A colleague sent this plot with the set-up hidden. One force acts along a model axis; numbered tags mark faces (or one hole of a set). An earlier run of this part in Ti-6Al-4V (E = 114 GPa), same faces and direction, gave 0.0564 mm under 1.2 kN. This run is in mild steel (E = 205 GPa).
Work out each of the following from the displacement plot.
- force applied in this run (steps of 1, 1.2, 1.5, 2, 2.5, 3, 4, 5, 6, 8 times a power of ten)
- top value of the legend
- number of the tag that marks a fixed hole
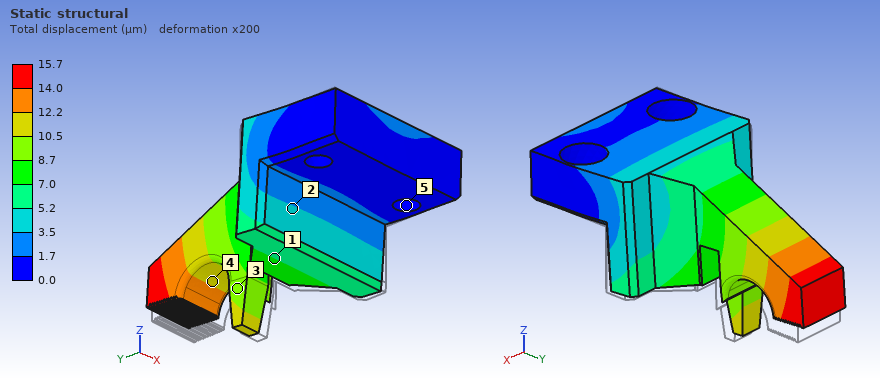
600 N
15.7 µm
5
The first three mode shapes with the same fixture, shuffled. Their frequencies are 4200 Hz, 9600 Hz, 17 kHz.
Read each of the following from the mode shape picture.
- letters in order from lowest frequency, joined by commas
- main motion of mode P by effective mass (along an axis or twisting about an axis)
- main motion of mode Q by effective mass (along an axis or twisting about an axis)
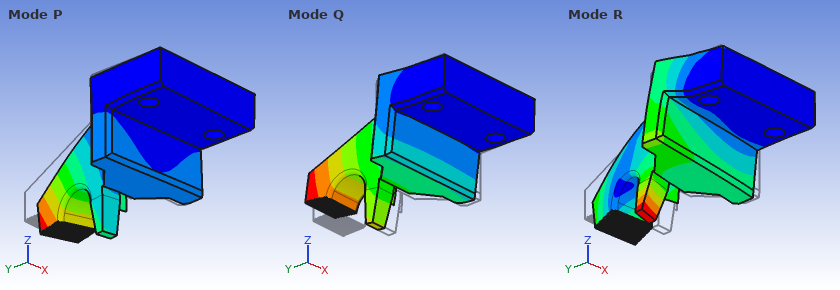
Q, P, R
along X
along Z
